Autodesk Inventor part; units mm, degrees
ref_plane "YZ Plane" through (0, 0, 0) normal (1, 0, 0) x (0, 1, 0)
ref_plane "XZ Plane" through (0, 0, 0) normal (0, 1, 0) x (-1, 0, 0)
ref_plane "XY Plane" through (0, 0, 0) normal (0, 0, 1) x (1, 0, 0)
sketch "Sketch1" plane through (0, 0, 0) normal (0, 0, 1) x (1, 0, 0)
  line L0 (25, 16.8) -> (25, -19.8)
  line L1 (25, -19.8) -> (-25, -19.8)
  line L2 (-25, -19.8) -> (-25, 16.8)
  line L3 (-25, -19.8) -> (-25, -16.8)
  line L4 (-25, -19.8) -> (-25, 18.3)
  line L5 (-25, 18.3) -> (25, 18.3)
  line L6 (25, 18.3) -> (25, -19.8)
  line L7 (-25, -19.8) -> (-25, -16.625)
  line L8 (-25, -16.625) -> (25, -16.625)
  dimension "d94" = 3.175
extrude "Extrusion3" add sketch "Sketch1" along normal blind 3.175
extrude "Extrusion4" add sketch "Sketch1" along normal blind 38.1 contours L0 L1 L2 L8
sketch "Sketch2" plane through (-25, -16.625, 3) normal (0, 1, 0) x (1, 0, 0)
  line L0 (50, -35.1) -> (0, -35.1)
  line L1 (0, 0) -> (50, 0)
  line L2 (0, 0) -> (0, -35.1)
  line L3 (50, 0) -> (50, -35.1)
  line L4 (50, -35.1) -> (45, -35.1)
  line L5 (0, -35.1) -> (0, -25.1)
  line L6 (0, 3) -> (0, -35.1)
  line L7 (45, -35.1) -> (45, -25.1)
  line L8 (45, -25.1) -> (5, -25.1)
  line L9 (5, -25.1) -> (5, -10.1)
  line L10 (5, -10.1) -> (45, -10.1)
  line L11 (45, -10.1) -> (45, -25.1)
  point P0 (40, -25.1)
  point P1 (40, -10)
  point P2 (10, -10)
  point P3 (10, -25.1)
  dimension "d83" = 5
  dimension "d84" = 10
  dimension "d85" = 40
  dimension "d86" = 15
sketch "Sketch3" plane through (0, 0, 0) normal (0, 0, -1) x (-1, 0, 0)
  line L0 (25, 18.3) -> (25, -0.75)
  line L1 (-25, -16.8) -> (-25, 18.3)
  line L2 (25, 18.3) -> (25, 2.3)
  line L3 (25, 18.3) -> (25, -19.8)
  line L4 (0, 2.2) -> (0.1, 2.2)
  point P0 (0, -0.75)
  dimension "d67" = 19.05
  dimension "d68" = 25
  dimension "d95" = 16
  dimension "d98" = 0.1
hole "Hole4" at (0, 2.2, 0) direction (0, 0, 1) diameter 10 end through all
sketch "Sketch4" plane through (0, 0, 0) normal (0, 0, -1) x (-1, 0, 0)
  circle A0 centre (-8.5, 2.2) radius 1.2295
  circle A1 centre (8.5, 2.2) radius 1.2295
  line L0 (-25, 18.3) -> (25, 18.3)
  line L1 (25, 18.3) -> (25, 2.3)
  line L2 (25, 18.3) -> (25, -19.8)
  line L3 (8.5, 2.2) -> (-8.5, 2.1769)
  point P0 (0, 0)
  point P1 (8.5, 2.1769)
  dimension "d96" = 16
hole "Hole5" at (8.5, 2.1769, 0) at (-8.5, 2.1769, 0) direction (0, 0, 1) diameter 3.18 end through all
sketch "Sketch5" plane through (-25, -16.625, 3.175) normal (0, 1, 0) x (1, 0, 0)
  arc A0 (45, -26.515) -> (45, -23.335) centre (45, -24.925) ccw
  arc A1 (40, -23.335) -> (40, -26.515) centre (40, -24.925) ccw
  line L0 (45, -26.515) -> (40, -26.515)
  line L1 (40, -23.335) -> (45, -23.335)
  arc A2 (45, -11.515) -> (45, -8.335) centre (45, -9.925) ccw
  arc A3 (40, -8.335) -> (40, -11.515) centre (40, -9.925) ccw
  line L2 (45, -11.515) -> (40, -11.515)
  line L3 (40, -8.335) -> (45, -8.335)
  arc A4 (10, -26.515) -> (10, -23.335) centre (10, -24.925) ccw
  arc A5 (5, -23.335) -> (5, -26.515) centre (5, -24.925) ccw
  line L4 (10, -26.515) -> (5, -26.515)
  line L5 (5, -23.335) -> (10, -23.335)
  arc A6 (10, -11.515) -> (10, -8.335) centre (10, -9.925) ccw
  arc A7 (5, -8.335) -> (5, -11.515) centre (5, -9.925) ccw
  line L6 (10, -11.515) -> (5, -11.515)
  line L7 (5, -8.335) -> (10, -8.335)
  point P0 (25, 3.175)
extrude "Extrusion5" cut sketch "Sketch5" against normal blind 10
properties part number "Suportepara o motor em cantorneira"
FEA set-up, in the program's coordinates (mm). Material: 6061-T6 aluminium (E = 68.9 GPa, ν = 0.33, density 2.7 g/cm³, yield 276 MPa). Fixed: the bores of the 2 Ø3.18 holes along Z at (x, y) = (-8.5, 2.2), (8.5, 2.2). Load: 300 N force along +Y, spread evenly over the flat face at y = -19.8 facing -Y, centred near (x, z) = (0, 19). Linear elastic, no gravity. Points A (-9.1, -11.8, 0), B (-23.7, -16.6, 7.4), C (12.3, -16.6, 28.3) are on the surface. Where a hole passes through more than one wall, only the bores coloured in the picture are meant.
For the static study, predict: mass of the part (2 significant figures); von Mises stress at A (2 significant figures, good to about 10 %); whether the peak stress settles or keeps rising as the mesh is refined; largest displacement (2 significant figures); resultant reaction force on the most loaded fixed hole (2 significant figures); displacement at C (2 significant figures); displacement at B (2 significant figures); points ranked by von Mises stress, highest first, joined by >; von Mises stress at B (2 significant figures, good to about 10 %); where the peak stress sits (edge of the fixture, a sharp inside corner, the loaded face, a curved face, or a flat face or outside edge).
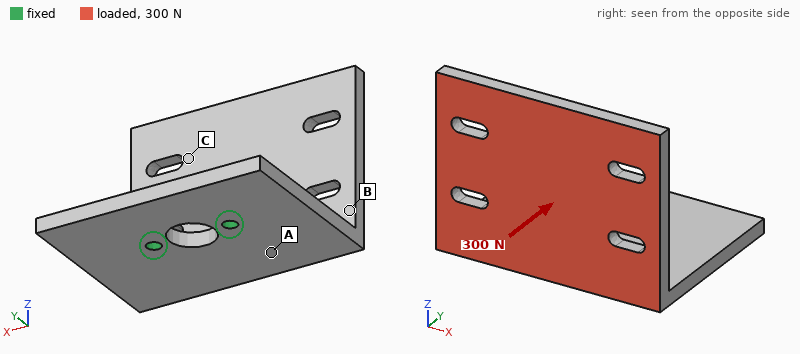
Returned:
30 g
53 MPa
keeps rising
0.67 mm
150 N
0.47 mm
0.14 mm
A > B > C
39 MPa
edge of the fixture
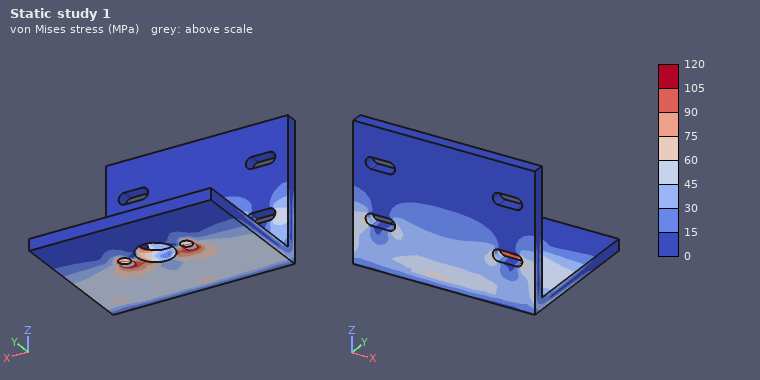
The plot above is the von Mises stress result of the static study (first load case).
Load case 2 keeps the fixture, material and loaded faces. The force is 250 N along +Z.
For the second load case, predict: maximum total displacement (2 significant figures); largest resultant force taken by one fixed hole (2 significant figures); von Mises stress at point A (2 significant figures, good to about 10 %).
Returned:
0.34 mm
130 N
21 MPa
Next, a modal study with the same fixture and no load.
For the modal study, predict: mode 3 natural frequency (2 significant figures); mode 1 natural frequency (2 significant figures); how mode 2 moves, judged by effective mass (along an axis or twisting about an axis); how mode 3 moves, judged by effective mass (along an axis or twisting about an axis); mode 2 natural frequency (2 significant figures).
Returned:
3000 Hz
970 Hz
along X
along Z
1700 Hz
